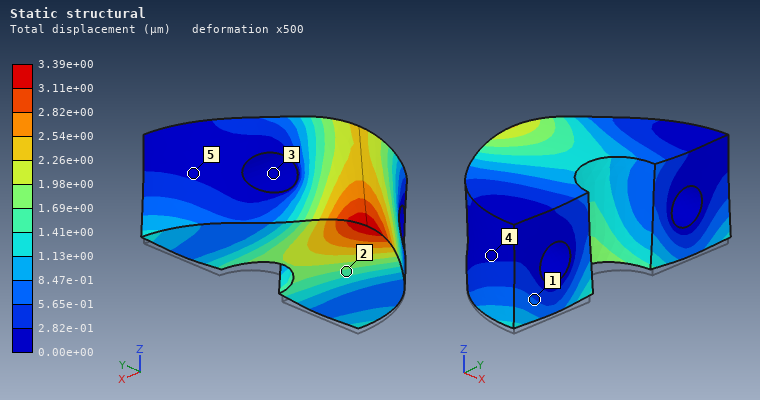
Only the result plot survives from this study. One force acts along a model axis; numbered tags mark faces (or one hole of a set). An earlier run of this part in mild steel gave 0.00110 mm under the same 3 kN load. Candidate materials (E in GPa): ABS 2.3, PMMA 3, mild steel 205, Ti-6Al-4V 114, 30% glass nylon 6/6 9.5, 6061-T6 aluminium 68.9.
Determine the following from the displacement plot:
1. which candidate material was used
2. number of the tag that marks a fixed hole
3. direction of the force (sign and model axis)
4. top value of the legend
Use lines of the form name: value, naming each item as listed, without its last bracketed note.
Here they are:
which candidate material was used: 6061-T6 aluminium
number of the tag that marks a fixed hole: 3
direction of the force: +Z
top value of the legend: 3.39e+00 µm
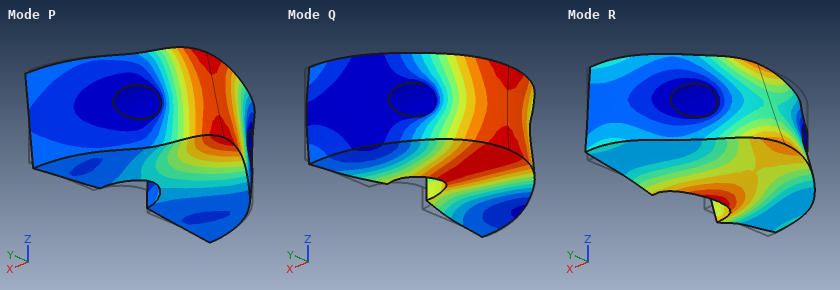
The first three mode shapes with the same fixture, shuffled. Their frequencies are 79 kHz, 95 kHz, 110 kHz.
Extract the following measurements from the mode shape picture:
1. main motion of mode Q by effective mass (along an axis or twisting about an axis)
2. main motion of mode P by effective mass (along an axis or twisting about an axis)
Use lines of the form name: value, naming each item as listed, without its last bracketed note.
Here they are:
main motion of mode Q by effective mass: along X
main motion of mode P by effective mass: along Z
